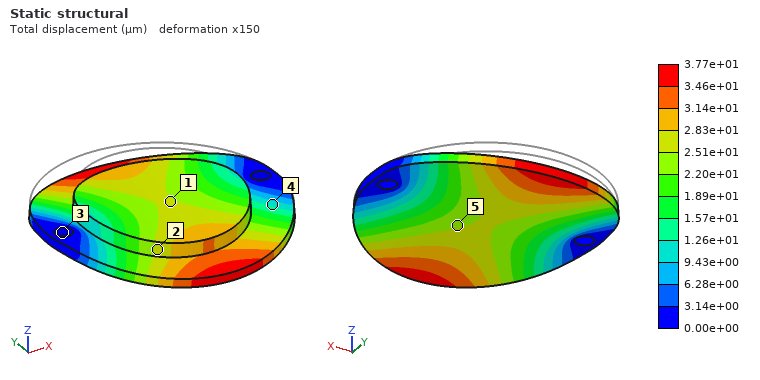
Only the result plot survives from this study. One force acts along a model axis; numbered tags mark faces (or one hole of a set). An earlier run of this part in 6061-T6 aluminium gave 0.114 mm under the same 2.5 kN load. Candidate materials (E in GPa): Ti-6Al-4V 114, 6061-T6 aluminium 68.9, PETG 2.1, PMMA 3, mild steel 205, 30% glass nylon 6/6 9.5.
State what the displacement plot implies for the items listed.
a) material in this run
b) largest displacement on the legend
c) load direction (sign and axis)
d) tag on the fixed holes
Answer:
mild steel
3.77e+01 µm
-Z
3
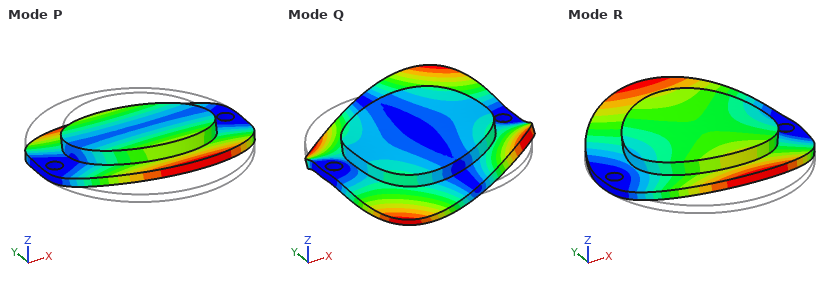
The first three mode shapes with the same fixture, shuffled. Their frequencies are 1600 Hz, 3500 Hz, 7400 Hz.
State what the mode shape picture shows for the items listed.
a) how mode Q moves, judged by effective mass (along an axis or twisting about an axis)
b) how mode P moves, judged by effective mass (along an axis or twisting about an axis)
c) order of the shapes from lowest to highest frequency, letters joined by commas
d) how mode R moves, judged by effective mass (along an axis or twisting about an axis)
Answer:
twisting about Y
twisting about X
P, R, Q
along Z
